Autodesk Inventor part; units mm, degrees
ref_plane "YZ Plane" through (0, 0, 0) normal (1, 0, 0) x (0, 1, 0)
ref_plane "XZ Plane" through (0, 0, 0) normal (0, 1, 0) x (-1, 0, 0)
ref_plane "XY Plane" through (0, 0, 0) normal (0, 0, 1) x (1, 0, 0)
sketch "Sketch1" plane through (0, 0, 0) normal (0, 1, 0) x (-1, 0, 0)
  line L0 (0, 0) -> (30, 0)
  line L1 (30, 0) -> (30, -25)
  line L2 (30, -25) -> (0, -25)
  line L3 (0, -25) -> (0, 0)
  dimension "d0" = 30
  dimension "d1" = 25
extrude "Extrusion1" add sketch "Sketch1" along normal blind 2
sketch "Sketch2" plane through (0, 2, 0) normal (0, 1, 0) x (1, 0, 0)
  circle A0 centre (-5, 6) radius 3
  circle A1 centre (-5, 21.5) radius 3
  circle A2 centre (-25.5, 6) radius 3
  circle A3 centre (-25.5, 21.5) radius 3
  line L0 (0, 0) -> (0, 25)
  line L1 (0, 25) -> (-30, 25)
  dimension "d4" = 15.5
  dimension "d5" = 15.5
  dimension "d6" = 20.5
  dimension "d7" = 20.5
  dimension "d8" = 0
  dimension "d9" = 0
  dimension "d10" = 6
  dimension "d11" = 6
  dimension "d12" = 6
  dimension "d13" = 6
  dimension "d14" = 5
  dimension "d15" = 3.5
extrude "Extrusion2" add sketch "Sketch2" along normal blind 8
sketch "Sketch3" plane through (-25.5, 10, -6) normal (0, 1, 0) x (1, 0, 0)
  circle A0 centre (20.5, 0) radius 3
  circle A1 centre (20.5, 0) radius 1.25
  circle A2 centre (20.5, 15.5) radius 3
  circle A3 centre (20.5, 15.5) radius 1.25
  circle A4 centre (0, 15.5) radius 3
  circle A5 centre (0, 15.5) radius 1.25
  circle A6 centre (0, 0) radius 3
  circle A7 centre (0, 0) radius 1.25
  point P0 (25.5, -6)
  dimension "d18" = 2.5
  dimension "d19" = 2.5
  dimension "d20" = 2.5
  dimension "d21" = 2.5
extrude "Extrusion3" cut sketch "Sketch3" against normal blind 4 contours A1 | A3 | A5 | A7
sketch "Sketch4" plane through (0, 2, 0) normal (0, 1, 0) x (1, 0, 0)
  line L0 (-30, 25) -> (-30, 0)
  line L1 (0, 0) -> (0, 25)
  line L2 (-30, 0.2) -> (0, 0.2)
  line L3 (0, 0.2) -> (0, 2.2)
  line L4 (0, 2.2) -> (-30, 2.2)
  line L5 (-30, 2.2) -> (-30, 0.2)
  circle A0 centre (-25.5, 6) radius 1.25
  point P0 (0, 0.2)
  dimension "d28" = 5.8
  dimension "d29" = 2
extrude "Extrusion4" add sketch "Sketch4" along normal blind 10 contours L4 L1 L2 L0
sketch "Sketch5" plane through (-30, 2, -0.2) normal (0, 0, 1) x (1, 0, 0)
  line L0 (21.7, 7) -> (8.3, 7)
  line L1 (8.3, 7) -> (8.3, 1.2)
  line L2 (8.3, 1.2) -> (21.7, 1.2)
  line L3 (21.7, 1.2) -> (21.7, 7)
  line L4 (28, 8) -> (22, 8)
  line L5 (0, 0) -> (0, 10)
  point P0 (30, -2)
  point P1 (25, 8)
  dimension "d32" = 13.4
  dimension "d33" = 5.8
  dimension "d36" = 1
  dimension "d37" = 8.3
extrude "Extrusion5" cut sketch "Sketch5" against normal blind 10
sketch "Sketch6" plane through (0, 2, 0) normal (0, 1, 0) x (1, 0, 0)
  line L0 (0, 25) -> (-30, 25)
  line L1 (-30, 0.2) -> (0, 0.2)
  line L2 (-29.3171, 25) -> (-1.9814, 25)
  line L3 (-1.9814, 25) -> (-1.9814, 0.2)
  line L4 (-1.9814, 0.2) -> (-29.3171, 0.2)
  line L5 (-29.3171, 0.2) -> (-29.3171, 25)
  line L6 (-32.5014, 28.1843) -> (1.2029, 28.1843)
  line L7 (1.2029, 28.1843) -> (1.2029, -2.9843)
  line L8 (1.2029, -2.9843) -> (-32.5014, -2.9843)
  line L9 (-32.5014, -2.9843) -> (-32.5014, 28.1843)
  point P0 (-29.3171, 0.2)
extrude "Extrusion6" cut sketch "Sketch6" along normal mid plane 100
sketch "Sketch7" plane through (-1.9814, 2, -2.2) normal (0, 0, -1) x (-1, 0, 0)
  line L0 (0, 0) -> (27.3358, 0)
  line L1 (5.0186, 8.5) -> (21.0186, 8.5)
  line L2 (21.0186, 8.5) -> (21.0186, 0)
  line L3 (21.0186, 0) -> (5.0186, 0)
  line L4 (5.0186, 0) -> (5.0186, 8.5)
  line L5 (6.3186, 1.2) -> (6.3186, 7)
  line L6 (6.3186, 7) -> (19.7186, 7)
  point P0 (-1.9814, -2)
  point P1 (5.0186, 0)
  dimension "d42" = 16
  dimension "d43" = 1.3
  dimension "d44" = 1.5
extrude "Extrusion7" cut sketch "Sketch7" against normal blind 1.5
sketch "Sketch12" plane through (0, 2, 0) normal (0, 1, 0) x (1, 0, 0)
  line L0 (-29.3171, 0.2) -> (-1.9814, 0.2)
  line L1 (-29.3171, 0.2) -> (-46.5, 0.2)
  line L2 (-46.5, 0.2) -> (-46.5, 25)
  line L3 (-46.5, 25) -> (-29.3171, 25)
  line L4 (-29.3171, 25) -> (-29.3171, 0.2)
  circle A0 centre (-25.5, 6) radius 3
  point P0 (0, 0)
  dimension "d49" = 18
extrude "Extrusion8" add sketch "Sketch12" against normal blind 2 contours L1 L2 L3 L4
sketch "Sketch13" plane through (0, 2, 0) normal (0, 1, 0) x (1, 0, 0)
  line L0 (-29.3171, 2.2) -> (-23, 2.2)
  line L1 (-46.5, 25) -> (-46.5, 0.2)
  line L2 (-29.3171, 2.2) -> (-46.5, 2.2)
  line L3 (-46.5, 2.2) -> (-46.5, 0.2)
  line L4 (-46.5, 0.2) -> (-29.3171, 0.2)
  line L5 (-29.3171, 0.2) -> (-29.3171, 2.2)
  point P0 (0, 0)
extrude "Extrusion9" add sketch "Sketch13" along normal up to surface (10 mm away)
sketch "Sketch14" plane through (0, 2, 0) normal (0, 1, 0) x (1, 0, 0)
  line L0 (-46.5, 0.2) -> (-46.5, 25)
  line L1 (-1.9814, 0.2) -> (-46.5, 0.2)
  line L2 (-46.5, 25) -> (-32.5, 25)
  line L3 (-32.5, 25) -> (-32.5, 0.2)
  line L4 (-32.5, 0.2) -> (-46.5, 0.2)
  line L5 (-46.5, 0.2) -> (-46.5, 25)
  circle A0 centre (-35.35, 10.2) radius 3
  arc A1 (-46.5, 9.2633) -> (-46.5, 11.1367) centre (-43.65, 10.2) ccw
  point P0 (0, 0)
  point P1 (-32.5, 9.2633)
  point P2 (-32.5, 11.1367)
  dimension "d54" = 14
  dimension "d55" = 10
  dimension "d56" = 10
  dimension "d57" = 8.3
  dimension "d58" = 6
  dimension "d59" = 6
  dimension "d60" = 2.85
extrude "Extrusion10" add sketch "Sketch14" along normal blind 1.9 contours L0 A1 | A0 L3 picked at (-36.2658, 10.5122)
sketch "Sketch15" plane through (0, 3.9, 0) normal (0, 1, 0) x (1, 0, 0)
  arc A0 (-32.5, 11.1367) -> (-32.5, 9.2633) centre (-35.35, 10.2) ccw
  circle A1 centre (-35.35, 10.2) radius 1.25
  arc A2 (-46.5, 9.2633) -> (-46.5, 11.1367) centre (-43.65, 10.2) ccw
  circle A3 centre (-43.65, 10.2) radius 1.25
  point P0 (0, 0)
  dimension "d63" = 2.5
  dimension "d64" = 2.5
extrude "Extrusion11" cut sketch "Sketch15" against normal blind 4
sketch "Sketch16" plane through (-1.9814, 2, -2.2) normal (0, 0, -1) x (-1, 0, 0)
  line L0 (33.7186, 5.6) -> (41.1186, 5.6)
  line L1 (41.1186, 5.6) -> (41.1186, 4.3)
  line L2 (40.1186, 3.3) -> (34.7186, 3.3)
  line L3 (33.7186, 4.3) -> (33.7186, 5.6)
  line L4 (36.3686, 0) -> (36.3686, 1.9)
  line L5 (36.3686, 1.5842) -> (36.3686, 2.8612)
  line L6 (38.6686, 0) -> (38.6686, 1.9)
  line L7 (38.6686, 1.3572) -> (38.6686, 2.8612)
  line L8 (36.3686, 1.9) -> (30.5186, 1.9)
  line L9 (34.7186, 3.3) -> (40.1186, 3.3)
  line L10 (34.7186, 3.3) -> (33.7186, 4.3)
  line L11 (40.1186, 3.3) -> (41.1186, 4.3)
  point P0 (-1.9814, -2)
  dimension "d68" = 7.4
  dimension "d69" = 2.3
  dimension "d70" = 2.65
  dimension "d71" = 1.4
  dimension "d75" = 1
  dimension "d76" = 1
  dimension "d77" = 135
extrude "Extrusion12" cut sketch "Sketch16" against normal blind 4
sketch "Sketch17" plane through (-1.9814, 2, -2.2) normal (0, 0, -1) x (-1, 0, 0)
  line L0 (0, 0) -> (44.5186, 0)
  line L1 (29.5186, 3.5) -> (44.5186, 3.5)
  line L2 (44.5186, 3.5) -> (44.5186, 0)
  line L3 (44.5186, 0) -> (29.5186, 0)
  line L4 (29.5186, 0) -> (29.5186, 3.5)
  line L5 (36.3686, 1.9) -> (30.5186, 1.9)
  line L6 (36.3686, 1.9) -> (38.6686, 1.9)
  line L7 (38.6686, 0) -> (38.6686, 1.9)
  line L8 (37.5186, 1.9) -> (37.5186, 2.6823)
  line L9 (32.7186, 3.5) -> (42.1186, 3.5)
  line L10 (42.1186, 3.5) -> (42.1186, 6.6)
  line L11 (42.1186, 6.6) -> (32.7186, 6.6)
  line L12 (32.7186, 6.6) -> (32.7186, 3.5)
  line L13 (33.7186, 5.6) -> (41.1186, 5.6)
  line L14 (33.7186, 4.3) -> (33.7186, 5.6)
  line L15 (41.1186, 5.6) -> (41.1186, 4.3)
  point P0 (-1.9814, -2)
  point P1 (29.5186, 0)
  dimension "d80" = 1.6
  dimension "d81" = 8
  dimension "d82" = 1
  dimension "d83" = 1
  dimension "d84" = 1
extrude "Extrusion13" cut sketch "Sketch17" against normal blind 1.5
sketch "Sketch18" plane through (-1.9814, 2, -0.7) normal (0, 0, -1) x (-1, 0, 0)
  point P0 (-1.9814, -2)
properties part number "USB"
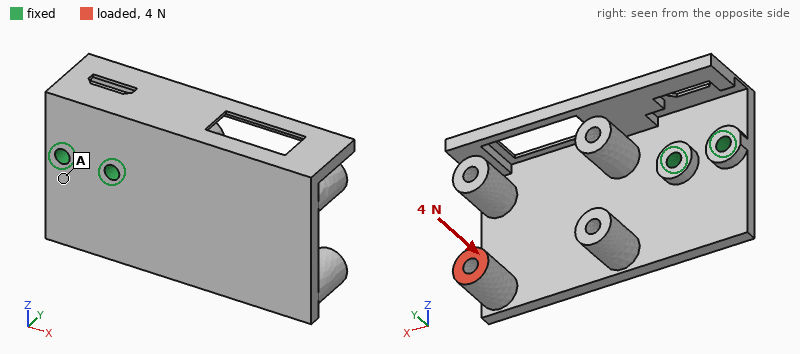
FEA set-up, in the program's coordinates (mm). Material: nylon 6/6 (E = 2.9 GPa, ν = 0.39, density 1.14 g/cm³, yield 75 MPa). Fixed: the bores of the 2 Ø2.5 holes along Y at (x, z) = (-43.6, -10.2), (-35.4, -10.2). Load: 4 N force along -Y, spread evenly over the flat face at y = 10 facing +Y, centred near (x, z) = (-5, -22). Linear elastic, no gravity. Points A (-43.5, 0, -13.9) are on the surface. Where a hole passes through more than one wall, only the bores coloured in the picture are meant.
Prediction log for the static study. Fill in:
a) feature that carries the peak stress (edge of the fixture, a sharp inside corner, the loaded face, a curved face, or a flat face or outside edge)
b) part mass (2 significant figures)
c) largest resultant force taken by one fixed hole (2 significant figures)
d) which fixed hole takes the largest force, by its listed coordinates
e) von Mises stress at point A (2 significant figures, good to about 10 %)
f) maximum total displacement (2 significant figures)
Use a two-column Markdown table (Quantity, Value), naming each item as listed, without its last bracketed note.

| Quantity | Value |
|---|---|
| feature that carries the peak stress | a flat face or outside edge |
| part mass | 4.1 g |
| largest resultant force taken by one fixed hole | 11 N |
| which fixed hole takes the largest force, by its listed coordinates | (-35.4, -10.2) |
| von Mises stress at point A | 0.79 MPa |
| maximum total displacement | 0.61 mm |
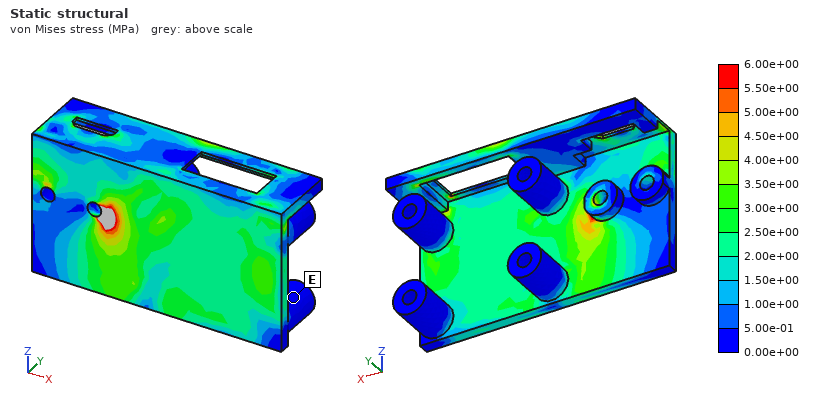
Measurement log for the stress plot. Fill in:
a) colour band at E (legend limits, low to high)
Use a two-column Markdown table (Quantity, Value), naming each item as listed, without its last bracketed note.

| Quantity | Value |
|---|---|
| colour band at E | 0.00e+00 to 5.00e-01 MPa |
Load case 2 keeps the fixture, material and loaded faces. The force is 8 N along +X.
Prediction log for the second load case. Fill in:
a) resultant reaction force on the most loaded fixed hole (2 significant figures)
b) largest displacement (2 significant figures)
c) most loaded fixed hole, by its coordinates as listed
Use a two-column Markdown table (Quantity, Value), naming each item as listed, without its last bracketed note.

| Quantity | Value |
|---|---|
| resultant reaction force on the most loaded fixed hole | 11 N |
| largest displacement | 0.53 mm |
| most loaded fixed hole, by its coordinates as listed | (-35.4, -10.2) |
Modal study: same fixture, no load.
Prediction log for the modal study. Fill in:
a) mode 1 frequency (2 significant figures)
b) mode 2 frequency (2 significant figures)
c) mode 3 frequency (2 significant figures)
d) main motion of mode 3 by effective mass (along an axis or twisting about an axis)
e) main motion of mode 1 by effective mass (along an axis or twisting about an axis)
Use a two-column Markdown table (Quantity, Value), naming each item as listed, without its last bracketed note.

| Quantity | Value |
|---|---|
| mode 1 frequency | 490 Hz |
| mode 2 frequency | 770 Hz |
| mode 3 frequency | 1800 Hz |
| main motion of mode 3 by effective mass | along Z |
| main motion of mode 1 by effective mass | along Y |
